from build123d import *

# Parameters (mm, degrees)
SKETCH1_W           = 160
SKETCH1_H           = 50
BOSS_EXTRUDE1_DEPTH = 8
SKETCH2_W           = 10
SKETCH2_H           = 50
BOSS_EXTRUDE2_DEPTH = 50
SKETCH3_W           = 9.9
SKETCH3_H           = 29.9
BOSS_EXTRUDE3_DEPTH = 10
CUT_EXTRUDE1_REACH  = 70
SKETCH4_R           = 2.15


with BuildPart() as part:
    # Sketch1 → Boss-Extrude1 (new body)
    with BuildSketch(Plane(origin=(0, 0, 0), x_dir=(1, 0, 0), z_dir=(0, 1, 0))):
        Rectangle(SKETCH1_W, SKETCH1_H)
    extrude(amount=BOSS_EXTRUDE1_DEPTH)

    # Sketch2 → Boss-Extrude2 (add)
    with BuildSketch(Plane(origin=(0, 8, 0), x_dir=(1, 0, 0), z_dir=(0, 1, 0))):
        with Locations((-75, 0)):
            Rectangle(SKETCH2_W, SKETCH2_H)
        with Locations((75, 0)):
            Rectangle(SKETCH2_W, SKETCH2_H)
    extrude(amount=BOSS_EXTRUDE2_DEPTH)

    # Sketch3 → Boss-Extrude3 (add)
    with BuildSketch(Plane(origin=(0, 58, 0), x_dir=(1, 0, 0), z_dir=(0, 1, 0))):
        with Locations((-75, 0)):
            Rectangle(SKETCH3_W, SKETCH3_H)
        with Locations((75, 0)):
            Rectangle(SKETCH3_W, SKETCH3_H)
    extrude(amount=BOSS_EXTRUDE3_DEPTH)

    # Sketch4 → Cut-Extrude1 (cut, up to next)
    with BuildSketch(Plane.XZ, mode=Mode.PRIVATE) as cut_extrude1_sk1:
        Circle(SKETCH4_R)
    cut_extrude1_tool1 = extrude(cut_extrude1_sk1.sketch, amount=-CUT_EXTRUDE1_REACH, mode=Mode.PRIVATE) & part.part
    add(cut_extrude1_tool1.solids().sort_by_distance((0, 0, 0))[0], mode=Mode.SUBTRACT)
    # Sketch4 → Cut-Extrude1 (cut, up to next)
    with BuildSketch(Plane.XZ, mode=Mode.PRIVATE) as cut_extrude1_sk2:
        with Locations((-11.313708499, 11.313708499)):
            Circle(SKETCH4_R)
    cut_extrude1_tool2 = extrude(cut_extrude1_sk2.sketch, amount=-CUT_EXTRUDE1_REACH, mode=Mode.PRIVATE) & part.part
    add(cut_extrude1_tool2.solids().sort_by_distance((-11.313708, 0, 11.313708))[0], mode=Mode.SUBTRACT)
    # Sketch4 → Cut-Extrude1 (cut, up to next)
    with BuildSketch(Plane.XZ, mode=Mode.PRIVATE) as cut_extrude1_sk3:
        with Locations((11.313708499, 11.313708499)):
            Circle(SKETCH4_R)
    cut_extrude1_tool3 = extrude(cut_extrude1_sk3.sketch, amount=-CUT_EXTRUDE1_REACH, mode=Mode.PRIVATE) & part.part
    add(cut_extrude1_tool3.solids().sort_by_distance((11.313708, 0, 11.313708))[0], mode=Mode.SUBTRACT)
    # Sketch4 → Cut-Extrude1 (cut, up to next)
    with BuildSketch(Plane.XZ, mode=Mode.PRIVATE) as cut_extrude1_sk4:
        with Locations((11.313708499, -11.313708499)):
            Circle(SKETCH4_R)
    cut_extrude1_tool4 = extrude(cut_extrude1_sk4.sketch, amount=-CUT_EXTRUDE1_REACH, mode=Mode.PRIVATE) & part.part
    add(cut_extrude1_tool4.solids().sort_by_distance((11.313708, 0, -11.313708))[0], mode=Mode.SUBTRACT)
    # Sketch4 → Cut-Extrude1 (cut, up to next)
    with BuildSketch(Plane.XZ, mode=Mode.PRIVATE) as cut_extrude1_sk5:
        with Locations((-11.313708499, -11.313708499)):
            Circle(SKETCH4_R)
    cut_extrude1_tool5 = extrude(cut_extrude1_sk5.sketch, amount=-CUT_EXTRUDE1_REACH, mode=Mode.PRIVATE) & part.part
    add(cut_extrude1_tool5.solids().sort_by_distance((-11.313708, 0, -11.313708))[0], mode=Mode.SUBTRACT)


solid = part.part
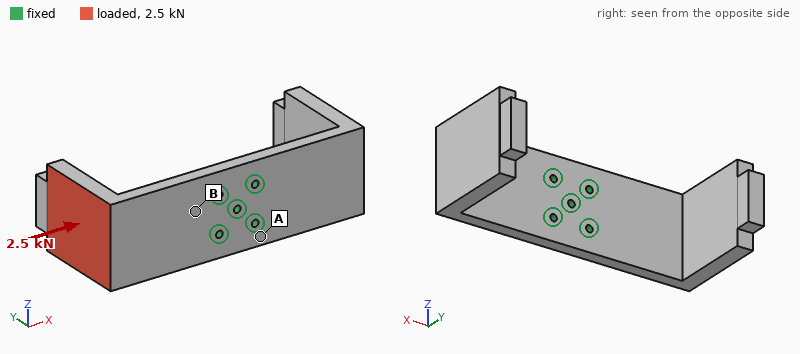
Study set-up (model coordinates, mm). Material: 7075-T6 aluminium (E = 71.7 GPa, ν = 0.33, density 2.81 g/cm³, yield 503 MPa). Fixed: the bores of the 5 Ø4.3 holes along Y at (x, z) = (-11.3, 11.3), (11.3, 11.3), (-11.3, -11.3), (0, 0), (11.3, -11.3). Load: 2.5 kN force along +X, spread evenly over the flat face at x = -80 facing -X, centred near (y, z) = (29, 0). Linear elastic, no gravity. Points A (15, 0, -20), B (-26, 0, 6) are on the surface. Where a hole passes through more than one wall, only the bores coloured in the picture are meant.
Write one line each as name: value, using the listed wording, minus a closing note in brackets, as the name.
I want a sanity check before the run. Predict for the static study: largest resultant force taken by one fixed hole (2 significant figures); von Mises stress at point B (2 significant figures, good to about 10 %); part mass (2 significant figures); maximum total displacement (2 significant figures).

largest resultant force taken by one fixed hole: 1.2 kN
von Mises stress at point B: 100 MPa
part mass: 340 g
maximum total displacement: 2.0 mm
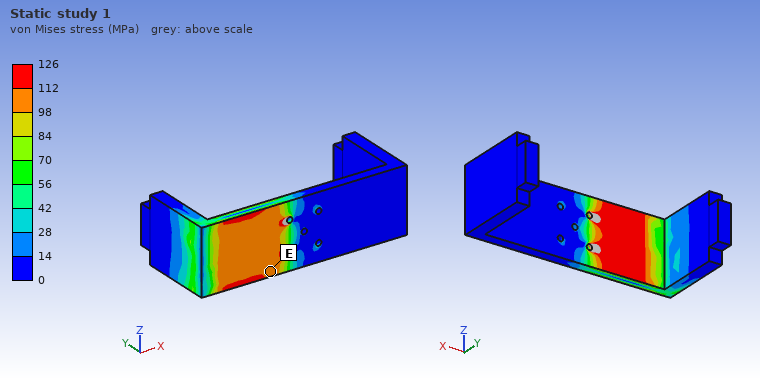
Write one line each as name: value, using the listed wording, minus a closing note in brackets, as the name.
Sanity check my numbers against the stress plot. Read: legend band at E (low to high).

legend band at E: 98 to 112 MPa
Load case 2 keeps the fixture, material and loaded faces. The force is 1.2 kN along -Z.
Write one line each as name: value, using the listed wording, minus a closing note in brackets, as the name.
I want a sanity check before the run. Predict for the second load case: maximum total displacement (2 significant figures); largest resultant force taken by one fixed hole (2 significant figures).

maximum total displacement: 0.46 mm
largest resultant force taken by one fixed hole: 2.5 kN
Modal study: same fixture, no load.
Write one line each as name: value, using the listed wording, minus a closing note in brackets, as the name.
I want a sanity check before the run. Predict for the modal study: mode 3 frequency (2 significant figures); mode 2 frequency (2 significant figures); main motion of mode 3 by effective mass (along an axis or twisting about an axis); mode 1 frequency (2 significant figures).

mode 3 frequency: 940 Hz
mode 2 frequency: 520 Hz
main motion of mode 3 by effective mass: twisting about Y
mode 1 frequency: 510 Hz
